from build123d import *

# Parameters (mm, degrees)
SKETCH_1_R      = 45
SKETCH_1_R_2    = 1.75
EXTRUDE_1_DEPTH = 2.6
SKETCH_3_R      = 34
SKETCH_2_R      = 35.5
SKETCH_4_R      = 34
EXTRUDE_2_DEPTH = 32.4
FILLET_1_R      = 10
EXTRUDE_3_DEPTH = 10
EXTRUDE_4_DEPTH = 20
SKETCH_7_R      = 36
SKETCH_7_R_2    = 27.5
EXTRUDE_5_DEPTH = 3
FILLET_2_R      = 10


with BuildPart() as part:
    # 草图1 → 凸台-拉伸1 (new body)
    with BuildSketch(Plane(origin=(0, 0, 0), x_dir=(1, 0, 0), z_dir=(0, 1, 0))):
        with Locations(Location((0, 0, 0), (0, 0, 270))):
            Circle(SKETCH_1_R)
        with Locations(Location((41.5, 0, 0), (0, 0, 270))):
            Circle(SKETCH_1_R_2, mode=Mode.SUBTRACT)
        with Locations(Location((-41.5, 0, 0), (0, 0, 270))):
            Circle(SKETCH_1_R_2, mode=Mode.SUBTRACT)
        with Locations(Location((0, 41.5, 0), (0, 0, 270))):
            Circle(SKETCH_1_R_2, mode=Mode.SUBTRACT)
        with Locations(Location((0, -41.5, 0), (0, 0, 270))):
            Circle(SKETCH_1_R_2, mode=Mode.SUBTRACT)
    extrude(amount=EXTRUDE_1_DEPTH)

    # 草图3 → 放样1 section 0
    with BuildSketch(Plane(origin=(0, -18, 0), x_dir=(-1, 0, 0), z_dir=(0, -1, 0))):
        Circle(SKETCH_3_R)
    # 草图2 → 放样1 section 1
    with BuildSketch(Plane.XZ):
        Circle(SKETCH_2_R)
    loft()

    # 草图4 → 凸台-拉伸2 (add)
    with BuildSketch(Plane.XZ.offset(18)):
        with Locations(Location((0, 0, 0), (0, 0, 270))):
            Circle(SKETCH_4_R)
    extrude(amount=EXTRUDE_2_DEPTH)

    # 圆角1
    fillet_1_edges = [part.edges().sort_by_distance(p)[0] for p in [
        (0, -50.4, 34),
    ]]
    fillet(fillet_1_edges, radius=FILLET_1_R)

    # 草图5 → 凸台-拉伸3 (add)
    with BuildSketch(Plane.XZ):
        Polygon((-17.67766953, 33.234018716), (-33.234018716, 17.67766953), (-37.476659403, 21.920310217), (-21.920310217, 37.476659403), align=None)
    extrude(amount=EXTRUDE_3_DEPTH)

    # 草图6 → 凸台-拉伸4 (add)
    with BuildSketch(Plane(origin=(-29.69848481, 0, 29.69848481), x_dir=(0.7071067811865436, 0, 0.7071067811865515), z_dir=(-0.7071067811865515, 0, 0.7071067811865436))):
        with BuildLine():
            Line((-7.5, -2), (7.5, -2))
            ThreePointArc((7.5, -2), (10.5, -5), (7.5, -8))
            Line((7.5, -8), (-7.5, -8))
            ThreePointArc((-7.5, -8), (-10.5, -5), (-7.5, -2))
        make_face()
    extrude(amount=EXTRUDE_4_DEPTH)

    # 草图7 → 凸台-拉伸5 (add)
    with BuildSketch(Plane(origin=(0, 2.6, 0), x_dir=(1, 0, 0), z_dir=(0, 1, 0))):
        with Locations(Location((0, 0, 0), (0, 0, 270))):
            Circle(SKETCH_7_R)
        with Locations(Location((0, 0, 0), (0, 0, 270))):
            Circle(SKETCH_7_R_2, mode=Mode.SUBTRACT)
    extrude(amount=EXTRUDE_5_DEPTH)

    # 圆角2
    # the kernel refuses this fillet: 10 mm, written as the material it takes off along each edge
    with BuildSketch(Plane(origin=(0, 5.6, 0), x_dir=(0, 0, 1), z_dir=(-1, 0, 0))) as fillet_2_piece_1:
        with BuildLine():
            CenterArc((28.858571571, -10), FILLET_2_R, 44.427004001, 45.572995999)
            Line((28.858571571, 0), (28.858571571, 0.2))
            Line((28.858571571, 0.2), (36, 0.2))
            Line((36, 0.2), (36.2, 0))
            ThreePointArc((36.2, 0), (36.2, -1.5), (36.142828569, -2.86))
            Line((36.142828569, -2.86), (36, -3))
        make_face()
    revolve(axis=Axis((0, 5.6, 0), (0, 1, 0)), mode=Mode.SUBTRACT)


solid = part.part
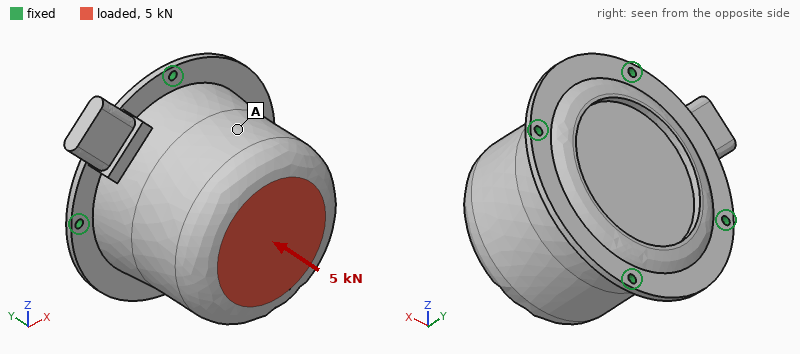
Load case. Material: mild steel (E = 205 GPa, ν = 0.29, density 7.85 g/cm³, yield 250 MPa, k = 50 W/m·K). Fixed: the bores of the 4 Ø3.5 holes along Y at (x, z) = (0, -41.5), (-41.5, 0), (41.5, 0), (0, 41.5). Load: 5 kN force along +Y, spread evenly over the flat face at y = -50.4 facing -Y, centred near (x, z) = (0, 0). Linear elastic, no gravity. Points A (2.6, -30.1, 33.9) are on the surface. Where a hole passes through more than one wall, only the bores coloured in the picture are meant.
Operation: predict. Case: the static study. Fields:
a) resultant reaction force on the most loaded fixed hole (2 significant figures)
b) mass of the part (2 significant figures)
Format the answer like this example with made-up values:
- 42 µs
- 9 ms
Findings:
- 1.3 kN
- 1.6 kg
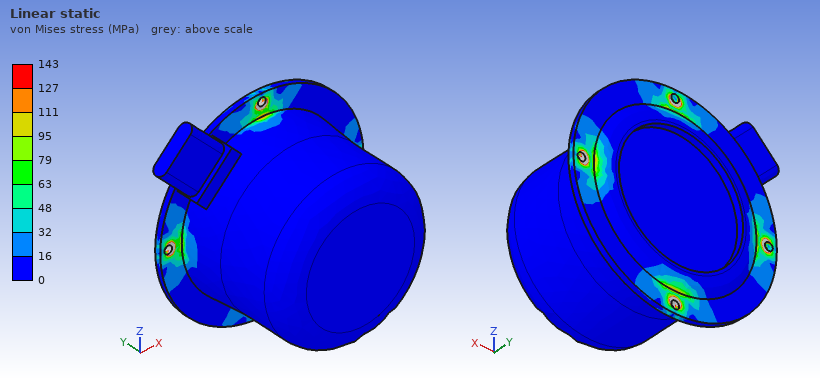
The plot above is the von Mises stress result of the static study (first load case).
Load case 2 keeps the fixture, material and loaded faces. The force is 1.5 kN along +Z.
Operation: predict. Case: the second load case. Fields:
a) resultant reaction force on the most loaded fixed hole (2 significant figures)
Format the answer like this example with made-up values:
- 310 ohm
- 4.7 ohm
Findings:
- 1.1 kN
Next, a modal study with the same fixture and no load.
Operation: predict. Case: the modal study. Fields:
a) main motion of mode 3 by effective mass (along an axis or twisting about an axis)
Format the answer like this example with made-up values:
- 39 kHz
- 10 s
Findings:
- along Y
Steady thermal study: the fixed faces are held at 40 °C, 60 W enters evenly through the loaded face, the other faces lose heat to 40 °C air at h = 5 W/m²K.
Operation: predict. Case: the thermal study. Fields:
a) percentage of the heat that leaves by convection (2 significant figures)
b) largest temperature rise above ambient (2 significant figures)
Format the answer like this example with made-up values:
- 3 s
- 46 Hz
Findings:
- 9.9 %
- 71 K
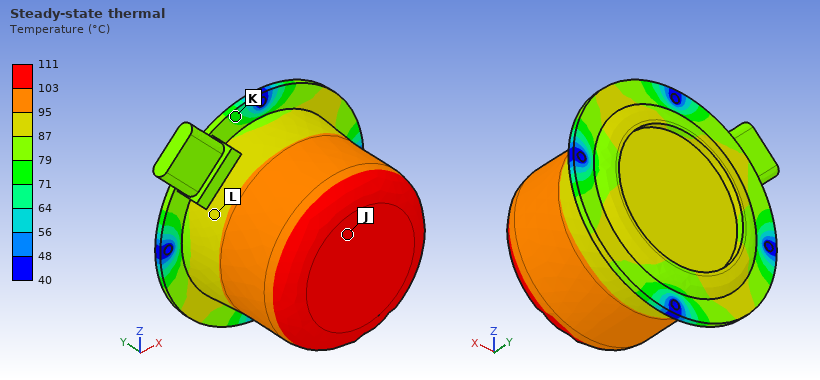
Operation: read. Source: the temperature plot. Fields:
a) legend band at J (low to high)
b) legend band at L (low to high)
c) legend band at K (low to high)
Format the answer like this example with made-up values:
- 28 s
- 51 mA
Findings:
- 103 to 111 °C
- 87 to 95 °C
- 71 to 79 °C
